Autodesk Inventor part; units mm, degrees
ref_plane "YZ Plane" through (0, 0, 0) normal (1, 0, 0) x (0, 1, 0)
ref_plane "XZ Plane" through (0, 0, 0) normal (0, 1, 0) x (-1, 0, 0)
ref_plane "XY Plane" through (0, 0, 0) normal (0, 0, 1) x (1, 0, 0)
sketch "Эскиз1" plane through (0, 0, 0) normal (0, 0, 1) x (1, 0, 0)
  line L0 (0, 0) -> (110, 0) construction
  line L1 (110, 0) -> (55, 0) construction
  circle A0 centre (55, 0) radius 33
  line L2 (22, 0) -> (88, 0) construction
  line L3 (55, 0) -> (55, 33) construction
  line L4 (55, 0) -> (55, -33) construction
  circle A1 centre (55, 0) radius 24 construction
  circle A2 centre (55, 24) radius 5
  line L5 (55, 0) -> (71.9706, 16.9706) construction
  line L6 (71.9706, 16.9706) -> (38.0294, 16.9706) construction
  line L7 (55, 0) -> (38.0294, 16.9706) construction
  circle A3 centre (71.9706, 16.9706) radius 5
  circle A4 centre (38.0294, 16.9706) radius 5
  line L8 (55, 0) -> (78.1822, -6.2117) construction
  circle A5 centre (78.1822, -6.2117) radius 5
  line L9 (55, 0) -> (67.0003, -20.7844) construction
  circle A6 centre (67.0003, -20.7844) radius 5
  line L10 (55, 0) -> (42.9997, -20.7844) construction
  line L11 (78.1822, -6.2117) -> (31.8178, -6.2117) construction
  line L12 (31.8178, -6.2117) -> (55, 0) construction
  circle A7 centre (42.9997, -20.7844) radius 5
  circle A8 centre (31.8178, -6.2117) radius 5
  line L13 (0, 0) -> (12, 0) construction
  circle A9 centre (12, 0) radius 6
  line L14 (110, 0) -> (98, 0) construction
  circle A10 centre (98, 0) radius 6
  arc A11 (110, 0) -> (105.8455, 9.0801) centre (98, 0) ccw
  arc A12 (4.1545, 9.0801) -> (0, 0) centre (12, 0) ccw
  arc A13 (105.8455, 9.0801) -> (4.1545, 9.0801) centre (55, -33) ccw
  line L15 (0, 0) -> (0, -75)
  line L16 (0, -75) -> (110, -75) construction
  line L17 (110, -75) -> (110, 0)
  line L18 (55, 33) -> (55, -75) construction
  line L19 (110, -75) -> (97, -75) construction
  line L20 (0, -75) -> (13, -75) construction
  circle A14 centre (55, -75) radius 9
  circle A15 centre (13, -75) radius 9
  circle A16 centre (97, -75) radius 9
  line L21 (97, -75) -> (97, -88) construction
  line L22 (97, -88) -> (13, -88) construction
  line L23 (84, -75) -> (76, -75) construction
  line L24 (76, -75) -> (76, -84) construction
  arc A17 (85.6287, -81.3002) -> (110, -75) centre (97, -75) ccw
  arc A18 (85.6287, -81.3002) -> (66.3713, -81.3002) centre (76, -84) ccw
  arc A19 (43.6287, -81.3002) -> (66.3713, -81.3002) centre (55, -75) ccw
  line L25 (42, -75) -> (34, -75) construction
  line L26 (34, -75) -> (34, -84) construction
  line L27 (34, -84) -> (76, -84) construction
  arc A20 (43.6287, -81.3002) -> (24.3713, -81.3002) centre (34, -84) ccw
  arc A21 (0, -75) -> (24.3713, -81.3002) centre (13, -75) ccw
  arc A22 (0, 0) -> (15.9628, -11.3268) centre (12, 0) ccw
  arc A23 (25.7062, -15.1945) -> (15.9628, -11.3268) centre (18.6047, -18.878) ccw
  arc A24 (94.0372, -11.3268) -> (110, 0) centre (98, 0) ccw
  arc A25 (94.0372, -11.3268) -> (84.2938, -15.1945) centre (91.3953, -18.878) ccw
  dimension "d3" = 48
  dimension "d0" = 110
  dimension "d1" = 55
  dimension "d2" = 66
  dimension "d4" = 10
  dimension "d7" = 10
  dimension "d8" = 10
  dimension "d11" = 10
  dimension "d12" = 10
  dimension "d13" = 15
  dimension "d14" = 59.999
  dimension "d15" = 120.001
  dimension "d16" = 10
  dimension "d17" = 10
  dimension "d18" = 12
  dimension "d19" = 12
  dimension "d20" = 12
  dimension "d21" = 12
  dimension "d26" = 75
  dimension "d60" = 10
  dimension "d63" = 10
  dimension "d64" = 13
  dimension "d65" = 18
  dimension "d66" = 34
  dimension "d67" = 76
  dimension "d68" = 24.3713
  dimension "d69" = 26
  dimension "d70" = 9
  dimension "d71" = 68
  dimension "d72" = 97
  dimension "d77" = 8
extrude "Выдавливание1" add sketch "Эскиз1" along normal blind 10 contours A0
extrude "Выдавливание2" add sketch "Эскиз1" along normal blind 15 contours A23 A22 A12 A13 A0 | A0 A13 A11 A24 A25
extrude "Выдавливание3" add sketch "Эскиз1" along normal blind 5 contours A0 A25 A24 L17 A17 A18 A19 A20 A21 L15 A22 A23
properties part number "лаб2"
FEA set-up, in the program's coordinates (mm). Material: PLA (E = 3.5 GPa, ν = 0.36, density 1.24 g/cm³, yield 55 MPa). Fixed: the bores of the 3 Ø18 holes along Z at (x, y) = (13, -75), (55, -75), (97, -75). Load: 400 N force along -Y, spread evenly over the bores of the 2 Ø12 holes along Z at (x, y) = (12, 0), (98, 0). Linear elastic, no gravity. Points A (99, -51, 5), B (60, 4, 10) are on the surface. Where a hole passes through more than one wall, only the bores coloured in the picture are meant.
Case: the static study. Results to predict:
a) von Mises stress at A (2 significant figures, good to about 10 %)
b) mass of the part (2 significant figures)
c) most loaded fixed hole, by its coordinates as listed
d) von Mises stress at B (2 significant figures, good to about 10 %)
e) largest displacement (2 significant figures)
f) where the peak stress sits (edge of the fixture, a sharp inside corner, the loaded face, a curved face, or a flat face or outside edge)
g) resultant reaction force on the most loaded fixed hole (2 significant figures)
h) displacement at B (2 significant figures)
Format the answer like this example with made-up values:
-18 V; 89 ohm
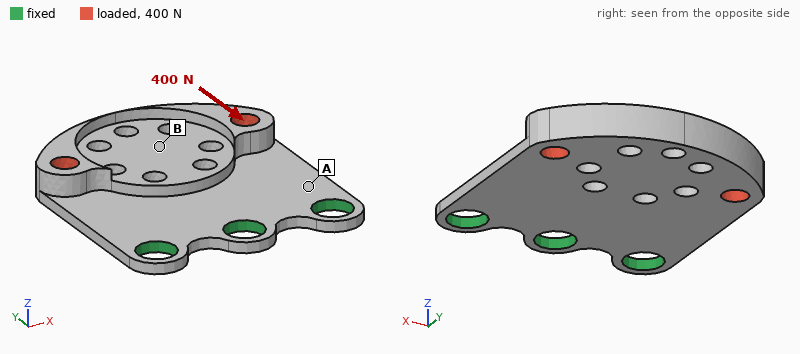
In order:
4.5 MPa; 96 g; (55, -75); 0.90 MPa; 1.7 mm; a flat face or outside edge; 160 N; 1.1 mm
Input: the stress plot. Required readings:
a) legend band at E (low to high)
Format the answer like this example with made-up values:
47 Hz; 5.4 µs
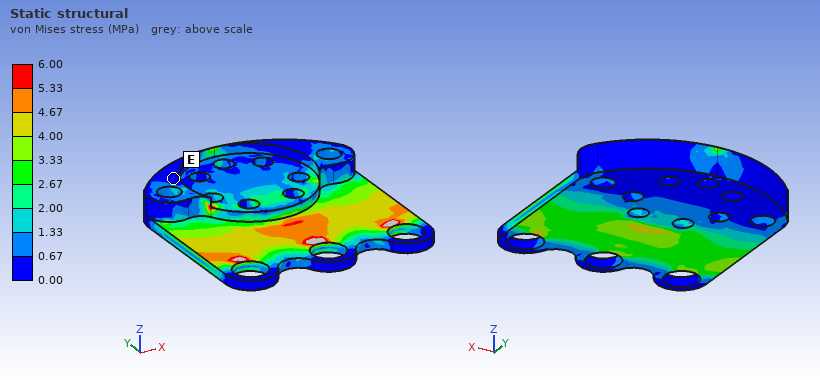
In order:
0.00 to 0.67 MPa
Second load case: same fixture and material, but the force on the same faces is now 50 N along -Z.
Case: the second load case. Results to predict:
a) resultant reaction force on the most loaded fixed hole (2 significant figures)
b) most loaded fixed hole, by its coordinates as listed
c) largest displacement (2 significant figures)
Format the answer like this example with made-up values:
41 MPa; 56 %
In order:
22 N; (55, -75); 2.0 mm
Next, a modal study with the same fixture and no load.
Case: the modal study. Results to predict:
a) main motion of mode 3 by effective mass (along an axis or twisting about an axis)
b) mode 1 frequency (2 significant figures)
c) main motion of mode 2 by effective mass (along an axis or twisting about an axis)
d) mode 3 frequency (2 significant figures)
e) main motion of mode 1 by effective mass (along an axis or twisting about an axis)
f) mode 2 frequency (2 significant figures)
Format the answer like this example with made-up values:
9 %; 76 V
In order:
along Z; 120 Hz; twisting about Y; 980 Hz; along Z; 380 Hz
